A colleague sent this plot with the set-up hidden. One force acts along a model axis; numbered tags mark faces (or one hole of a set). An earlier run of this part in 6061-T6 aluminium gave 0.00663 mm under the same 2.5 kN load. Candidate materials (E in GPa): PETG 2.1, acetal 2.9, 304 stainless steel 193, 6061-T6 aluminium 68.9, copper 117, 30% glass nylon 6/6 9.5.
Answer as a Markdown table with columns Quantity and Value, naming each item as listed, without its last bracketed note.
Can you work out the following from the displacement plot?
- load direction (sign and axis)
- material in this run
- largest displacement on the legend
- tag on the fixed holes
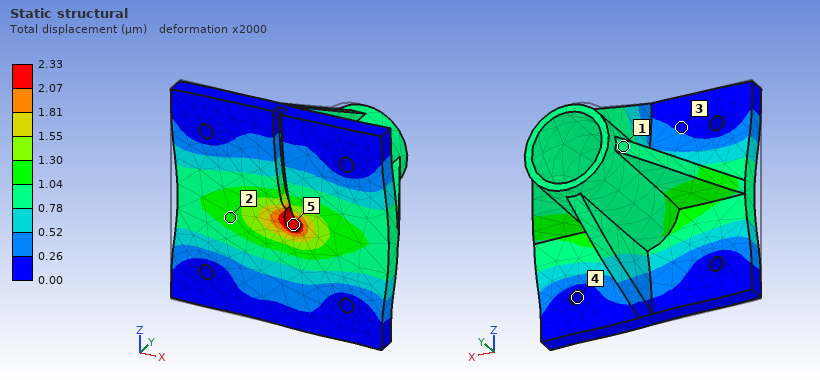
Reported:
| Quantity | Value |
|---|---|
| load direction | +X |
| material in this run | 304 stainless steel |
| largest displacement on the legend | 2.33 µm |
| tag on the fixed holes | 4 |
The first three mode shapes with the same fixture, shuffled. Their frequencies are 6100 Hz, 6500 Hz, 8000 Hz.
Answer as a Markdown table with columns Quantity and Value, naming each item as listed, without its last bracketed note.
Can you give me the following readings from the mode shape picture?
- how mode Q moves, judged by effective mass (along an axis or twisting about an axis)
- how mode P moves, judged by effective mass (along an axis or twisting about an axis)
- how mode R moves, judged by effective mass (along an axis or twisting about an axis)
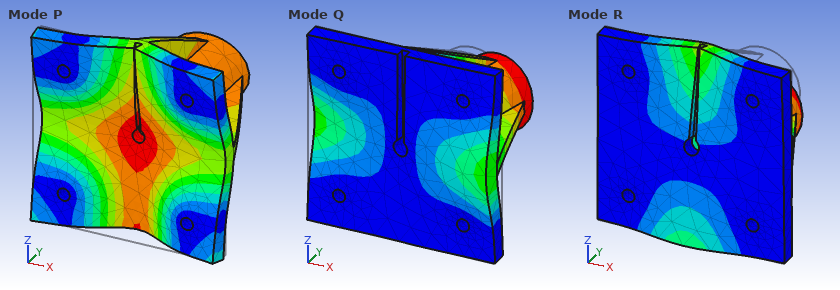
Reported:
| Quantity | Value |
|---|---|
| how mode Q moves, judged by effective mass | along X |
| how mode P moves, judged by effective mass | along Y |
| how mode R moves, judged by effective mass | along Z |
